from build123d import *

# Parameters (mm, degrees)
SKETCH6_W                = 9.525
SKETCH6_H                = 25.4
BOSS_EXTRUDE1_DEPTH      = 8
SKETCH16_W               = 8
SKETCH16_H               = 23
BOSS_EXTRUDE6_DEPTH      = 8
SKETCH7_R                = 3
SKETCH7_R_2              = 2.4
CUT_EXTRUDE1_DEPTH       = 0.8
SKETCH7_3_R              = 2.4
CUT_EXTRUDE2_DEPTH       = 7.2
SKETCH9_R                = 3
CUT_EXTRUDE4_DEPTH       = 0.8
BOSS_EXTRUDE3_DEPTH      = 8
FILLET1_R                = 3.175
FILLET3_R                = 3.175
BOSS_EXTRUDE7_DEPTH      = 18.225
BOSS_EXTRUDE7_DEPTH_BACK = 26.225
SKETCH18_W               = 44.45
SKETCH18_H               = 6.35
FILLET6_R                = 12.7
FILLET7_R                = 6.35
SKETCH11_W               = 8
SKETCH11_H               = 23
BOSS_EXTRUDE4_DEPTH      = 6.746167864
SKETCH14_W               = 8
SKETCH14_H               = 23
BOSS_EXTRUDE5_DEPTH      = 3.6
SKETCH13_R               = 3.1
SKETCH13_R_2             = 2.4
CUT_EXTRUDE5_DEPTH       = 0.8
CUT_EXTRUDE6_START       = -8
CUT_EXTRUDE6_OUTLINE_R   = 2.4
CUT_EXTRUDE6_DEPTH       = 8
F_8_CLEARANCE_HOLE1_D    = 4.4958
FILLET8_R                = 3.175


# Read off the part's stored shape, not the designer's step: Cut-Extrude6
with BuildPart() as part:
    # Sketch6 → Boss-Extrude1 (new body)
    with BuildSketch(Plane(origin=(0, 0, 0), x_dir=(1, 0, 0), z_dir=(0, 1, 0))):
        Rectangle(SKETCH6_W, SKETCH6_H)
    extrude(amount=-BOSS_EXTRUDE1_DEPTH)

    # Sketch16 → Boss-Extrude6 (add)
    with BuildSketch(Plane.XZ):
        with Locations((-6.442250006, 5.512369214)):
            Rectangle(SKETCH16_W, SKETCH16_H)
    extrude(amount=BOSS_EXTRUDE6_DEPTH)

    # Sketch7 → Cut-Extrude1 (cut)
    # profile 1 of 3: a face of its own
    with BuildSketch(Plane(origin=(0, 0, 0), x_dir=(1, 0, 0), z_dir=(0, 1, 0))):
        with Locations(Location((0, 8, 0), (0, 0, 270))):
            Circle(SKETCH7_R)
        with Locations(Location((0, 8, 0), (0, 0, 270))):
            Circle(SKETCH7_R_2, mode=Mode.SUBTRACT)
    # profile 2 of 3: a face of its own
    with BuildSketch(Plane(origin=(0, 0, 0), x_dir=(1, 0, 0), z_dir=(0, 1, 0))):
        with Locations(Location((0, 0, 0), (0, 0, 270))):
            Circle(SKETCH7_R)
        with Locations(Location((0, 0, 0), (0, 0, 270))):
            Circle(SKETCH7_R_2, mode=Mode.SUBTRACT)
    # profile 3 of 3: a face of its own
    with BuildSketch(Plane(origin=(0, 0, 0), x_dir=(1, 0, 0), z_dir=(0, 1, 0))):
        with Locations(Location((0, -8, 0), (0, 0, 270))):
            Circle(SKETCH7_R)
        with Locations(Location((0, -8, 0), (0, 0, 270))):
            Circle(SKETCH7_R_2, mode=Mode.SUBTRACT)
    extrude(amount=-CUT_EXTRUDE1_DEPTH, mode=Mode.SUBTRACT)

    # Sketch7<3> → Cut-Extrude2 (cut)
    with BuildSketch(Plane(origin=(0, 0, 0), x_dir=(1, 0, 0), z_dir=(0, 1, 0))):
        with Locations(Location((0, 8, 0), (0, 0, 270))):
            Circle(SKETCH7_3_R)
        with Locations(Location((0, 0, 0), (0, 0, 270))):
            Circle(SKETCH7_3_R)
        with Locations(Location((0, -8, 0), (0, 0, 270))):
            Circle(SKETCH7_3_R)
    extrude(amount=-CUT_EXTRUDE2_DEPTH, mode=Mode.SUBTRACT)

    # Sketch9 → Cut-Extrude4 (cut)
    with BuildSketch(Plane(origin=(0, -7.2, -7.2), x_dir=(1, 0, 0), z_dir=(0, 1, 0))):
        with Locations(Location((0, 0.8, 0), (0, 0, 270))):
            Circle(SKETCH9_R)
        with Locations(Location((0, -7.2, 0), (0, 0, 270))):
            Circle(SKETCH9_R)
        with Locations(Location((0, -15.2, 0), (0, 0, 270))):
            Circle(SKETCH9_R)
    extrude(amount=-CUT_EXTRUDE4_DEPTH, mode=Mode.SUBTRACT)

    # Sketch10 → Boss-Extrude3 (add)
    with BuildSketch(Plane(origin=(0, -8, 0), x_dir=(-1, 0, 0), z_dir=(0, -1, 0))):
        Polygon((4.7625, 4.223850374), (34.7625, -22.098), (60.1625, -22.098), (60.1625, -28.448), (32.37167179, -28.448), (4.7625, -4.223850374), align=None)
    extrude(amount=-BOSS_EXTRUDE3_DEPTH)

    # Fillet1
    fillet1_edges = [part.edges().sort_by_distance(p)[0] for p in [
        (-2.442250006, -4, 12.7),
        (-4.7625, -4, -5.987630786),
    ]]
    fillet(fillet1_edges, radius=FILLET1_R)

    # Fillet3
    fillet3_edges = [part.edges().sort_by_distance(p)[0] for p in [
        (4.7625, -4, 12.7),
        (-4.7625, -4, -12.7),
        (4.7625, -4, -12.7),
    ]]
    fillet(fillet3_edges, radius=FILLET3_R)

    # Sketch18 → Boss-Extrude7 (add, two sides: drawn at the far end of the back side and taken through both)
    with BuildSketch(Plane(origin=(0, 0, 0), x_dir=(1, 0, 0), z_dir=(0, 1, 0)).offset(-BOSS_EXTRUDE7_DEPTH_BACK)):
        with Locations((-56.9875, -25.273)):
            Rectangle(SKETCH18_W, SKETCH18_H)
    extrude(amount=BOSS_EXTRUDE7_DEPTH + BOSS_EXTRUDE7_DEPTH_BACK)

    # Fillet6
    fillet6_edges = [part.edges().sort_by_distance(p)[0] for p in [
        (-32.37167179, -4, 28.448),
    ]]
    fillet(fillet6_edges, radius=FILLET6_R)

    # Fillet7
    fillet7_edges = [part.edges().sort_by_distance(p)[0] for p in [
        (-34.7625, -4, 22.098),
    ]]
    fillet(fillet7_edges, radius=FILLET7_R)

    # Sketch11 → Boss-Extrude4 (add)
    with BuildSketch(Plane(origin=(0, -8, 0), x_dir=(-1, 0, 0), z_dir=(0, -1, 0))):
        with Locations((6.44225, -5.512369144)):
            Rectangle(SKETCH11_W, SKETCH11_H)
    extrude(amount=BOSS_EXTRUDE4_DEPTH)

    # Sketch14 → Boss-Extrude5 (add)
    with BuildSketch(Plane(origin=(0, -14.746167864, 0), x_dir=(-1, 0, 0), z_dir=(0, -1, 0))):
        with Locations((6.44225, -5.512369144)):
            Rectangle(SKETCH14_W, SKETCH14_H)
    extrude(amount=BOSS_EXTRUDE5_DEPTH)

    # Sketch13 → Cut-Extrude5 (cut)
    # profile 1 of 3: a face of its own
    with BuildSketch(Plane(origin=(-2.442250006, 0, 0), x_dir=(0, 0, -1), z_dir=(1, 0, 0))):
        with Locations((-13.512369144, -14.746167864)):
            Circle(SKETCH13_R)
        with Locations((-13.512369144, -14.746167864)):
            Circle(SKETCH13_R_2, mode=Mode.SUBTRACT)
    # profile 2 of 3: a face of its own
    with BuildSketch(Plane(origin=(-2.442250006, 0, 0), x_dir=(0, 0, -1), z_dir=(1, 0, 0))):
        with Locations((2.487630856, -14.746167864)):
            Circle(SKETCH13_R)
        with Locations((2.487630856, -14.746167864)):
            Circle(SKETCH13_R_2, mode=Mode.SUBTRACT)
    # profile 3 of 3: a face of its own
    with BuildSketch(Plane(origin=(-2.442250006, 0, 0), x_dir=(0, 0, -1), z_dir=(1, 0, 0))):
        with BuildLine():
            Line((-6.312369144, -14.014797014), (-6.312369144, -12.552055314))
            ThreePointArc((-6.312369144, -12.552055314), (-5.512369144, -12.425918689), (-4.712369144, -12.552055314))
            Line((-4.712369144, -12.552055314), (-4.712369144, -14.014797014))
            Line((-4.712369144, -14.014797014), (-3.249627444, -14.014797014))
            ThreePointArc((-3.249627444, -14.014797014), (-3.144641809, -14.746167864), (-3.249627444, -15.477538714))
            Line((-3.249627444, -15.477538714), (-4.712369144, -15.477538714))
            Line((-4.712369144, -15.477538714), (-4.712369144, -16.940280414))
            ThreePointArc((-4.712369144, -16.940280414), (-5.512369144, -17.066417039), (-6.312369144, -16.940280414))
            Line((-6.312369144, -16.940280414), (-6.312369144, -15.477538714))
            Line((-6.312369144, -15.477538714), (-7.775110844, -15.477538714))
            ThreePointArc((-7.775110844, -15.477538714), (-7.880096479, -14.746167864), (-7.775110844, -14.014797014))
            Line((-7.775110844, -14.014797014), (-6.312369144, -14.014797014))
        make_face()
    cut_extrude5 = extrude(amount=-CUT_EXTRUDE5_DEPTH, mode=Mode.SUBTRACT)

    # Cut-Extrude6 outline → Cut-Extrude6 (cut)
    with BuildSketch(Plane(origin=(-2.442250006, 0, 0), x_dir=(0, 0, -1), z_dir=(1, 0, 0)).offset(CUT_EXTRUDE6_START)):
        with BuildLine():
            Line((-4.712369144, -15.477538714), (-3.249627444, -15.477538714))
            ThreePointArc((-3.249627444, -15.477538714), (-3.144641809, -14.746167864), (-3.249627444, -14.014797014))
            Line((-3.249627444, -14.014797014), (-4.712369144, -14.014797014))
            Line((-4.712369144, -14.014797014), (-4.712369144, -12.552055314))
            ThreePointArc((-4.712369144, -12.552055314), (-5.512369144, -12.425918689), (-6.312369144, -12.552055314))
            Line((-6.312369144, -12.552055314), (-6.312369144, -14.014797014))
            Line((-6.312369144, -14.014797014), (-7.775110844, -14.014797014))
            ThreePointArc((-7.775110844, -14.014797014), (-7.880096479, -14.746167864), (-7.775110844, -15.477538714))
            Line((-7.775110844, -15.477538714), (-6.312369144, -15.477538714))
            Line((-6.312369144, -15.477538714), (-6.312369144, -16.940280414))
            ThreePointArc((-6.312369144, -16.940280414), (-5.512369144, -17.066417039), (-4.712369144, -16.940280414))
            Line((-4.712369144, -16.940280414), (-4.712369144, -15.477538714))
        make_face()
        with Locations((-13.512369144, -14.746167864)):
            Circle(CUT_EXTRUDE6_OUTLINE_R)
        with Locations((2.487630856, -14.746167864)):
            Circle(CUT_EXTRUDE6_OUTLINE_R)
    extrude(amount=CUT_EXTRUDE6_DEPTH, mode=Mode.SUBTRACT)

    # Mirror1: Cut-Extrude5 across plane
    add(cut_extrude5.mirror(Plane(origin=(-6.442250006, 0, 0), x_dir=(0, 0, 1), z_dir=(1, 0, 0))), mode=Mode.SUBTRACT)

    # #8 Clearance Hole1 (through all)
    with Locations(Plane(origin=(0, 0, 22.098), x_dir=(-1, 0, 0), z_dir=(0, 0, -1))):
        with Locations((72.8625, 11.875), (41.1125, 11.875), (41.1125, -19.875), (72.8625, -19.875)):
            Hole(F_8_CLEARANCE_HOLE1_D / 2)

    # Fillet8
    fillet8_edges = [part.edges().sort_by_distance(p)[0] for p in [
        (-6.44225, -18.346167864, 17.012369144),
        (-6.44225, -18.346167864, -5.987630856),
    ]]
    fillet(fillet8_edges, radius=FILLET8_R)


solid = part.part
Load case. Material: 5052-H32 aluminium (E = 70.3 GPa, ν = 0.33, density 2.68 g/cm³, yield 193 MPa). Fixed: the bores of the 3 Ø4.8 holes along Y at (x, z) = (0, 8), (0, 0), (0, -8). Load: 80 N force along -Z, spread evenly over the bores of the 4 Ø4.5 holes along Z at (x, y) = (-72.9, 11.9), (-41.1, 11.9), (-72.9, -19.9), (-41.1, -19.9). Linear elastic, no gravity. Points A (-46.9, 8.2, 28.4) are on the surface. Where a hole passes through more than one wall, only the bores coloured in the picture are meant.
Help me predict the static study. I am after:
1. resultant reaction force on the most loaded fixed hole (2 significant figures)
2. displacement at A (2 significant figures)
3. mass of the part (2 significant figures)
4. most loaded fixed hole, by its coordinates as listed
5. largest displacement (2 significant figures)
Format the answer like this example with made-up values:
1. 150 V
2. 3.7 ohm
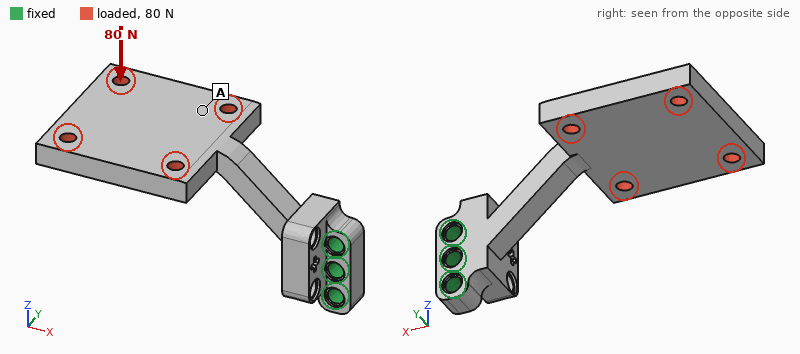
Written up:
1. 360 N
2. 0.23 mm
3. 48 g
4. (0, 8)
5. 0.48 mm
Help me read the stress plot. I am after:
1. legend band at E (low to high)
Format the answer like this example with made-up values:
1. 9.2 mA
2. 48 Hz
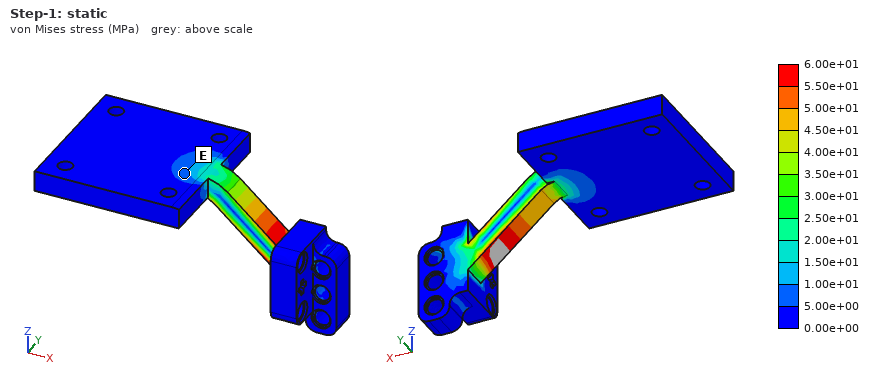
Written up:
1. 5.00e+00 to 1.00e+01 MPa
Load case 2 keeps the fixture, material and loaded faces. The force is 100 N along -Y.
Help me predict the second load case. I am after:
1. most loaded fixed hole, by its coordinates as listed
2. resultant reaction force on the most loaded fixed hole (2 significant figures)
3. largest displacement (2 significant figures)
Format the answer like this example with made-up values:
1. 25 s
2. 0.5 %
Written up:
1. (0, 8)
2. 140 N
3. 0.53 mm
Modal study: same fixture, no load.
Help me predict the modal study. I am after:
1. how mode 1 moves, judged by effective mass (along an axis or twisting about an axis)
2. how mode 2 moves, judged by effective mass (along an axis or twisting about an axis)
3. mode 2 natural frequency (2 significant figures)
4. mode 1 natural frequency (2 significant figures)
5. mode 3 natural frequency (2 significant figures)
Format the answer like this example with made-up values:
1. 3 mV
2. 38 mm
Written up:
1. along Z
2. along Y
3. 450 Hz
4. 420 Hz
5. 1200 Hz
